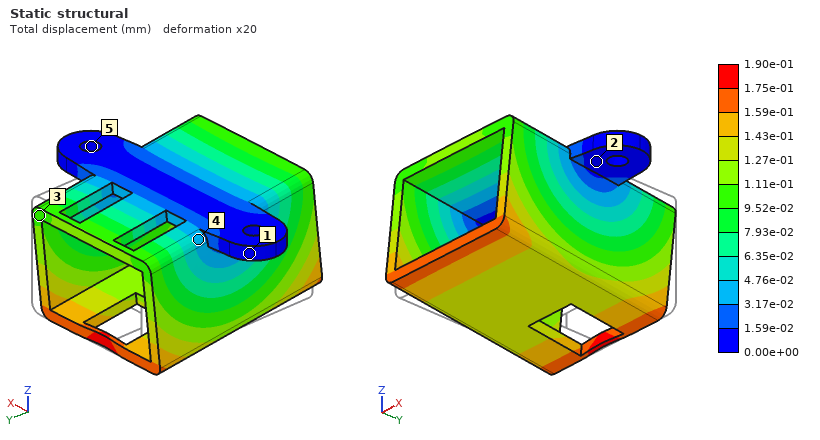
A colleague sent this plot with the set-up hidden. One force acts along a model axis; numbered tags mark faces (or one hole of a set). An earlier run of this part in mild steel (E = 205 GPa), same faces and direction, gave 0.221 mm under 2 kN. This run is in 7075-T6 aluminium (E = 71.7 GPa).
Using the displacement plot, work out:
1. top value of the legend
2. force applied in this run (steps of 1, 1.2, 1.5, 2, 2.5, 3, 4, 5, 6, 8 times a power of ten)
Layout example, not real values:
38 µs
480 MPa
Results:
1.90e-01 mm
600 N
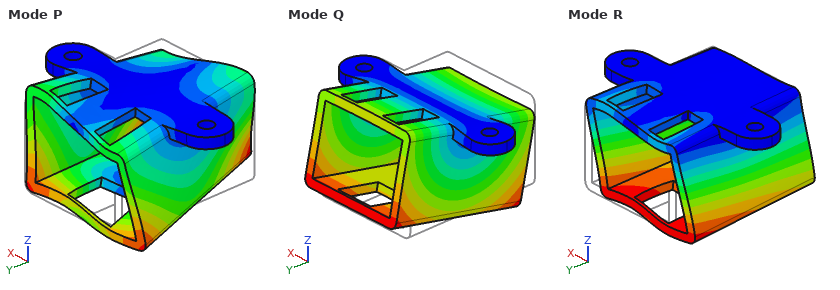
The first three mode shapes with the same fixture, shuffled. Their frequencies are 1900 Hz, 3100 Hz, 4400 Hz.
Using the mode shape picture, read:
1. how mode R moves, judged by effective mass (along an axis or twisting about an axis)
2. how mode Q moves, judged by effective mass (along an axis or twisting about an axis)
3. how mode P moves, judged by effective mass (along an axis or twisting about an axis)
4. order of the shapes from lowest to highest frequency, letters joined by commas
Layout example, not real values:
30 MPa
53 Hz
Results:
along X
along Y
twisting about Z
Q, R, P
